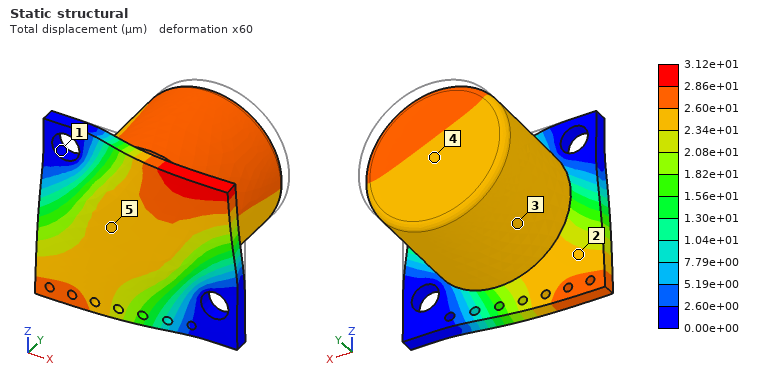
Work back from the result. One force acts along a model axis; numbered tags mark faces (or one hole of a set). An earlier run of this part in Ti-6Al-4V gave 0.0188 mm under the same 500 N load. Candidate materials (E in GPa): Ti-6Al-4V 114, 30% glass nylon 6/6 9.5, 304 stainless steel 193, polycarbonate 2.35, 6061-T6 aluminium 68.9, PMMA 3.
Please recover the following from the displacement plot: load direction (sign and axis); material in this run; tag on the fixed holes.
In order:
-Y
6061-T6 aluminium
1
